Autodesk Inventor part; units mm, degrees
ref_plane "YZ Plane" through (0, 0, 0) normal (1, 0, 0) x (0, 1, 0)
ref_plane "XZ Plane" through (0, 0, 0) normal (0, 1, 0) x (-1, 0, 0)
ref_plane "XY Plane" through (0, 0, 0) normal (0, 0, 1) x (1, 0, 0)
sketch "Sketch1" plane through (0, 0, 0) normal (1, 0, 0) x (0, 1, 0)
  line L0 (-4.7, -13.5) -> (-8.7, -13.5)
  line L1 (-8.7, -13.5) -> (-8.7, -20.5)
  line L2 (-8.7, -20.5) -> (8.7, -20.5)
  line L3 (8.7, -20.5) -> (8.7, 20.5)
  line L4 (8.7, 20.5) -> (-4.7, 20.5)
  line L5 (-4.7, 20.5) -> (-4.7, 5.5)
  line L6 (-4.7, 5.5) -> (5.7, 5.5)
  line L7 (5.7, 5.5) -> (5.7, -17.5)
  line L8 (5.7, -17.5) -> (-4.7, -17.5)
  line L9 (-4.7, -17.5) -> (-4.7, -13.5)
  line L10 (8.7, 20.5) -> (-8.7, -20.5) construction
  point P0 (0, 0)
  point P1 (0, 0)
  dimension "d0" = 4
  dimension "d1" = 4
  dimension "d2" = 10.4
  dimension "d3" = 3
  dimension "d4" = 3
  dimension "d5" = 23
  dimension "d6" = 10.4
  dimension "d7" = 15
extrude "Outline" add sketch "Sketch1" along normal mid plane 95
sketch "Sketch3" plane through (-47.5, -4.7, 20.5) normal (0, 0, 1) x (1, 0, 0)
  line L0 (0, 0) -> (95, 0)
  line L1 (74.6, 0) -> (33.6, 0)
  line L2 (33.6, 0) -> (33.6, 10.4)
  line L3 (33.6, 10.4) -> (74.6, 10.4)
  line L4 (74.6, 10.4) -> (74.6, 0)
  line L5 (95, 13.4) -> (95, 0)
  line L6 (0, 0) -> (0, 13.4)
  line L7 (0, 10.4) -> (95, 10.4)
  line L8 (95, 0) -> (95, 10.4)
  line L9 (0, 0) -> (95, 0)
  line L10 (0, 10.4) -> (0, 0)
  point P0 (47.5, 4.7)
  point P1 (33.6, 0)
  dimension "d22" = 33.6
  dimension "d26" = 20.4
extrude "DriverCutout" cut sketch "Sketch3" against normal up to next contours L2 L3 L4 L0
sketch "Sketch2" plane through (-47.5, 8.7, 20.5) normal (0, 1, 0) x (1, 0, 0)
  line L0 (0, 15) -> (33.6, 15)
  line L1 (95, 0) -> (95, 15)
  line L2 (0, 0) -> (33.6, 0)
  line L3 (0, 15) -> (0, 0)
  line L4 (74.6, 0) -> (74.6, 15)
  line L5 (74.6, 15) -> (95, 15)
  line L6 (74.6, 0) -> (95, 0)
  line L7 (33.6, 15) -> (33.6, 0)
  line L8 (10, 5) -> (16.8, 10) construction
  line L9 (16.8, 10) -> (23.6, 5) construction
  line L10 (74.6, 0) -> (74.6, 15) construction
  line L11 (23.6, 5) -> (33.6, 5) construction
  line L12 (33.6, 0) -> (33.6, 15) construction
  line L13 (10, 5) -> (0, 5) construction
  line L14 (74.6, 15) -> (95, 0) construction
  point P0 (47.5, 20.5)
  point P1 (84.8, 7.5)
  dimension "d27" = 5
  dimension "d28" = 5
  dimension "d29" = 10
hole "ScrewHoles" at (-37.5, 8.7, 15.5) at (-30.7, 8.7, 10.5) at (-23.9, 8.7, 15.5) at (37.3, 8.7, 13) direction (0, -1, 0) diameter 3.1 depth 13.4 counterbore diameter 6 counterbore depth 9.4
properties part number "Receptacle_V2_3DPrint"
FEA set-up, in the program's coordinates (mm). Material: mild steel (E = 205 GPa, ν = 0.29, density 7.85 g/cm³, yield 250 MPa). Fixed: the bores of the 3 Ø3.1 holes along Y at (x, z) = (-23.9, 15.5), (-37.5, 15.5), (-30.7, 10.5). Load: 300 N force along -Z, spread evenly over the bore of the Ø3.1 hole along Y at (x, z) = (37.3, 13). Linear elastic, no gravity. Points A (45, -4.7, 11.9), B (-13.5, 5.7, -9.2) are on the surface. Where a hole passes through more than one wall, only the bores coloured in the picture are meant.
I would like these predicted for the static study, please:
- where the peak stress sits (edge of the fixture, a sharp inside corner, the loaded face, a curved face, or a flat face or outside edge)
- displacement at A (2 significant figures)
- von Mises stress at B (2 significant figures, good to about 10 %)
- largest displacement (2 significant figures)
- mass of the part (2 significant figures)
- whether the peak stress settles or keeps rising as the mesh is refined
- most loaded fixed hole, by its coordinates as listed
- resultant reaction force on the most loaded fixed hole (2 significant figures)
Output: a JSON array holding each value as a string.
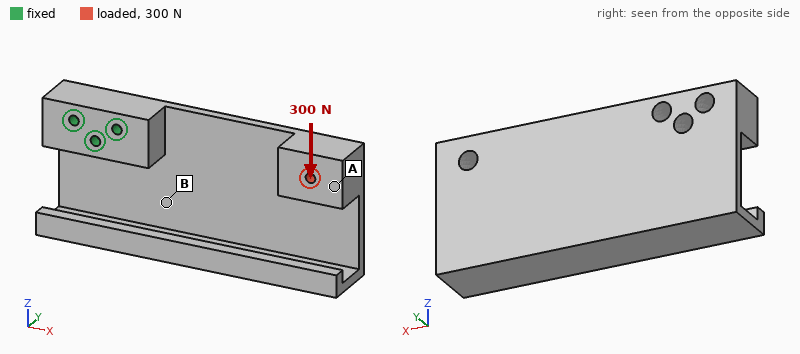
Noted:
["edge of the fixture", "0.090 mm", "16 MPa", "0.11 mm", "190 g", "keeps rising", "(-23.9, 15.5)", "1.2 kN"]
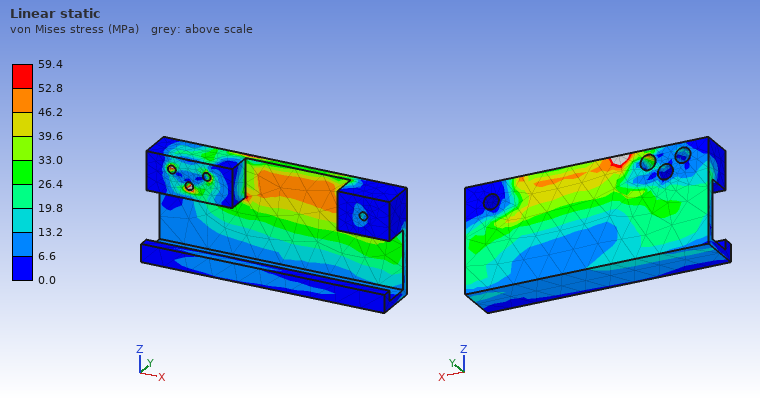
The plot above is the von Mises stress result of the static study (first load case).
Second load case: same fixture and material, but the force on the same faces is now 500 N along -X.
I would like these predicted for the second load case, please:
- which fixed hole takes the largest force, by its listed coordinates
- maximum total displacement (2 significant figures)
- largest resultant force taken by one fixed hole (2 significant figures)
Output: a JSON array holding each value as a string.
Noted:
["(-30.7, 10.5)", "0.21 mm", "300 N"]
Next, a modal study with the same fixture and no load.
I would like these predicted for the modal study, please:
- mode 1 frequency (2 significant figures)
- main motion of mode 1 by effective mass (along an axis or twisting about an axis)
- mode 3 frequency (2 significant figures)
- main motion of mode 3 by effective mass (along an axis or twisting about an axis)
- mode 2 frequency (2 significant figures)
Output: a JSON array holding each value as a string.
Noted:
["530 Hz", "along Y", "1800 Hz", "along Z", "970 Hz"]
